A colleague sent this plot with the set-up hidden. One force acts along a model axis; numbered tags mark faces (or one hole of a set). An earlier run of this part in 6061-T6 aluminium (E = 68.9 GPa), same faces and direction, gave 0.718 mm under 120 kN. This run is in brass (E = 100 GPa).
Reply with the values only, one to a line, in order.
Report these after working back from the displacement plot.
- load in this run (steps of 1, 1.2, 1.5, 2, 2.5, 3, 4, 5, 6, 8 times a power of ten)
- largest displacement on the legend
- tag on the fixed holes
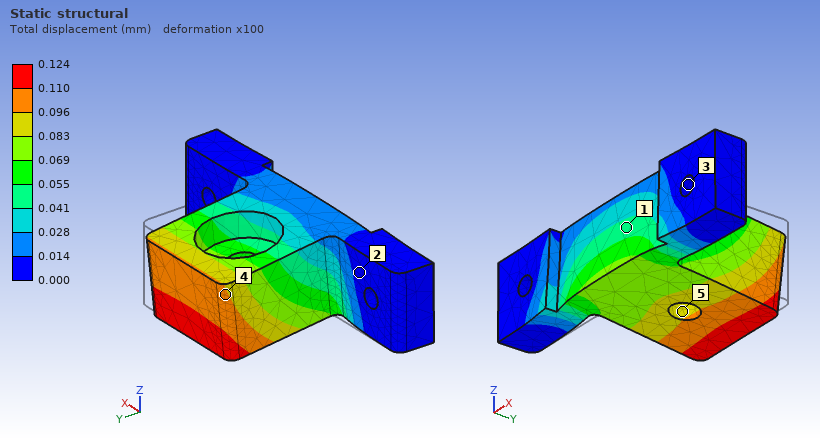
30 kN
0.124 mm
3
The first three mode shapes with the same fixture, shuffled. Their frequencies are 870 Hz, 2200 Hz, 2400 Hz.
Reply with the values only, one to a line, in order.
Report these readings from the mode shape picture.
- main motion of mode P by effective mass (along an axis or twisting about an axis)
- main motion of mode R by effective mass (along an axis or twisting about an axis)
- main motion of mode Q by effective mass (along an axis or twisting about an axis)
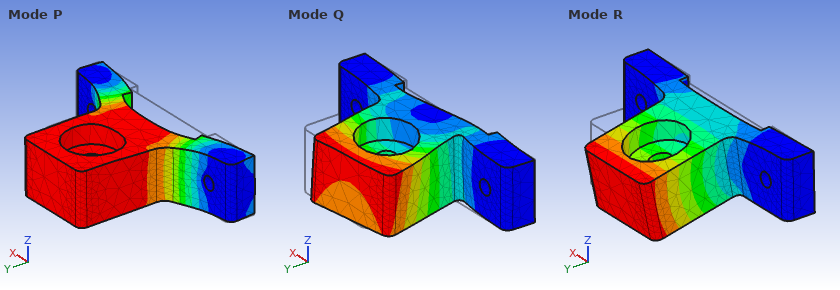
along Y
along Z
along X
